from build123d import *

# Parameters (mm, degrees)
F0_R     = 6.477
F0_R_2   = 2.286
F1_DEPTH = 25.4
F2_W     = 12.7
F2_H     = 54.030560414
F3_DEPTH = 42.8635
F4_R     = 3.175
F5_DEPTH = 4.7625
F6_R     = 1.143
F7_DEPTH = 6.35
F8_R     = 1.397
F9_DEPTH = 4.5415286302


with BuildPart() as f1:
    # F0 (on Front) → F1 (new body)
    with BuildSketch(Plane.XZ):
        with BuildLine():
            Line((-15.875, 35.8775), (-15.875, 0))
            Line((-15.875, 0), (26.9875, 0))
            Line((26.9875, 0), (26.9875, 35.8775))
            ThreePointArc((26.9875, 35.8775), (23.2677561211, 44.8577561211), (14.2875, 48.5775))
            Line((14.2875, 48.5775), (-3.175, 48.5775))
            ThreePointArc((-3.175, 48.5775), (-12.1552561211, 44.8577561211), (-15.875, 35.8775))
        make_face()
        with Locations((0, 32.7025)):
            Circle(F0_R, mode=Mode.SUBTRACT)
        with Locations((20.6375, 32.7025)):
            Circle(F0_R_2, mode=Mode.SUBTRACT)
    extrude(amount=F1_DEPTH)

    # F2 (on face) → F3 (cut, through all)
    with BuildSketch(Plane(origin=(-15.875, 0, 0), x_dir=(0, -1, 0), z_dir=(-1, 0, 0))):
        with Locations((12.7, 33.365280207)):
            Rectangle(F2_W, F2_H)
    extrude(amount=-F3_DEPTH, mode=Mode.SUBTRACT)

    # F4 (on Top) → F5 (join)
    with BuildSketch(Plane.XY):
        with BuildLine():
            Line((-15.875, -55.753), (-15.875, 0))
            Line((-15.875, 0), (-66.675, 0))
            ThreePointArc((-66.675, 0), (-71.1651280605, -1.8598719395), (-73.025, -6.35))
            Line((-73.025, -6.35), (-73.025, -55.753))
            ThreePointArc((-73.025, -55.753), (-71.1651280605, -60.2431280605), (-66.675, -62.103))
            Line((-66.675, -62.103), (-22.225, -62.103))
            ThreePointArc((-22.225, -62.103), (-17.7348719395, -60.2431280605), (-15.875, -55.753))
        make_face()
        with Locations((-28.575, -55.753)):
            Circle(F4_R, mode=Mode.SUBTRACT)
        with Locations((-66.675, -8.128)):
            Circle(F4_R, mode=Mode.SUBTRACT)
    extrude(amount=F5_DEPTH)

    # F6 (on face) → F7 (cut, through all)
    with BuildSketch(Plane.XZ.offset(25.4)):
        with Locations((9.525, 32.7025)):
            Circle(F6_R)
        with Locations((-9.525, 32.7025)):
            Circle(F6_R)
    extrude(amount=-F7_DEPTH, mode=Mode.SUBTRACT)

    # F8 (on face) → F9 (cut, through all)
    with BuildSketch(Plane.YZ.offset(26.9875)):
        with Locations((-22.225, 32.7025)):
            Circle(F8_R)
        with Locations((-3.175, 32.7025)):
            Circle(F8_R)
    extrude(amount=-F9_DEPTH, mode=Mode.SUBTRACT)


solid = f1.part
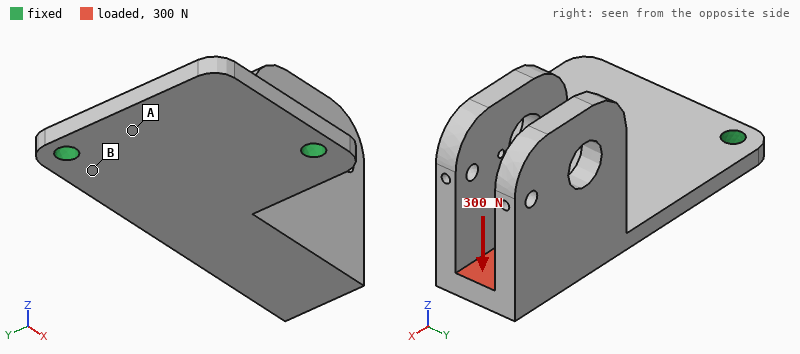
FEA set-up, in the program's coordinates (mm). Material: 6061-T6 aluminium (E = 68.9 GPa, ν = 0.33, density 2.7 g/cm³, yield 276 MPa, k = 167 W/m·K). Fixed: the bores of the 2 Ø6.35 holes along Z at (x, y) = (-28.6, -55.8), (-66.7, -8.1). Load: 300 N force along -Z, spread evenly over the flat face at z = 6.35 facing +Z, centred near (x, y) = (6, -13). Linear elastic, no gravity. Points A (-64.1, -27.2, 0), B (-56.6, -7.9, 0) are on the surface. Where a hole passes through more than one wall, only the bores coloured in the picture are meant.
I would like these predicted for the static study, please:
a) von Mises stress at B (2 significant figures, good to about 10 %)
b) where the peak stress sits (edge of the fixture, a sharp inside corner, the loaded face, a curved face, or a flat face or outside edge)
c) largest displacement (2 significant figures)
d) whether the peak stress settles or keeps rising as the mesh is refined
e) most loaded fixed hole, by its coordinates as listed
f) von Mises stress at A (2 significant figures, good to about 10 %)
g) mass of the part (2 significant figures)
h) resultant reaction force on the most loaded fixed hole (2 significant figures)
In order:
54 MPa
edge of the fixture
1.2 mm
keeps rising
(-28.6, -55.8)
13 MPa
120 g
270 N
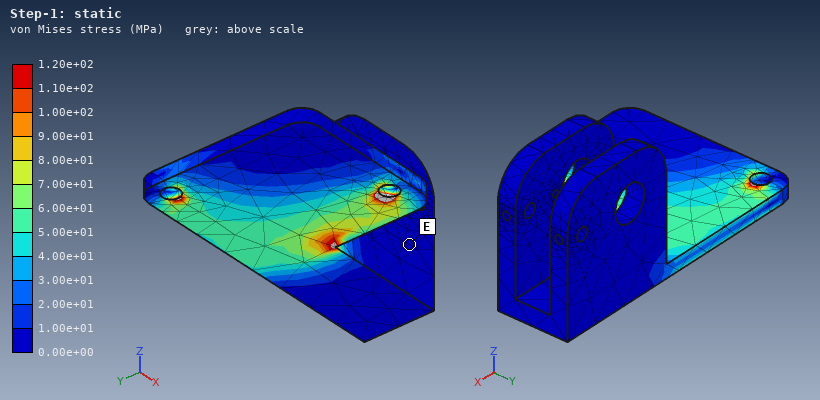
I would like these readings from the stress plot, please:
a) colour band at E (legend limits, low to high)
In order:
0.00e+00 to 1.00e+01 MPa
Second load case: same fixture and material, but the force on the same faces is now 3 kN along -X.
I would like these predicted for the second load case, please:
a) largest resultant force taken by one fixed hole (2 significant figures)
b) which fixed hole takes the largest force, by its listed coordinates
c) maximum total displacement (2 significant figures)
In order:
2.4 kN
(-66.7, -8.1)
1.2 mm
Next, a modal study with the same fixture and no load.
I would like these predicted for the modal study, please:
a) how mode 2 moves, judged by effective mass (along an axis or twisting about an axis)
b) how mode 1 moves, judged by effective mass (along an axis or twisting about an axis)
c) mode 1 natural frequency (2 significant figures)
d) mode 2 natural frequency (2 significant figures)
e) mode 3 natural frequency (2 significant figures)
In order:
along Y
along Z
330 Hz
790 Hz
1800 Hz
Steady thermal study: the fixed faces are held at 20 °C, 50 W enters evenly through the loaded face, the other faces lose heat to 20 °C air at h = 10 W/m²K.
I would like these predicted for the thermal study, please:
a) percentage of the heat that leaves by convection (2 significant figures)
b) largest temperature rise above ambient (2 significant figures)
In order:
17 %
79 K
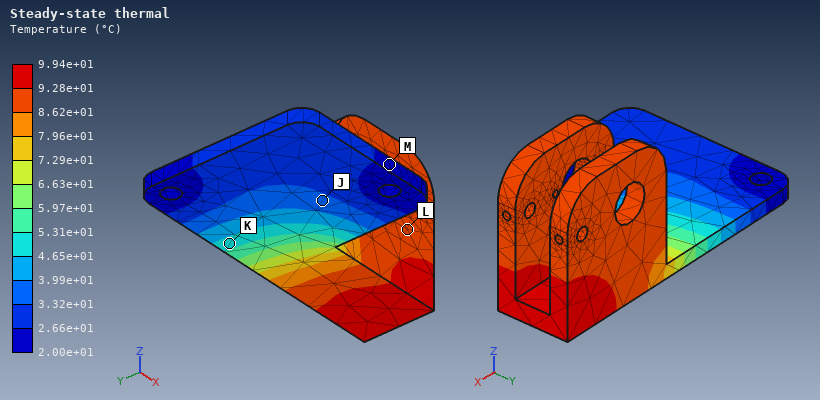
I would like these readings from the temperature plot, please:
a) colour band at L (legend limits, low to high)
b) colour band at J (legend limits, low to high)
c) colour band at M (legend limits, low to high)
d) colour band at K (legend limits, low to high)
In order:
8.62e+01 to 9.28e+01 °C
3.32e+01 to 3.99e+01 °C
2.00e+01 to 2.66e+01 °C
4.65e+01 to 5.31e+01 °C
